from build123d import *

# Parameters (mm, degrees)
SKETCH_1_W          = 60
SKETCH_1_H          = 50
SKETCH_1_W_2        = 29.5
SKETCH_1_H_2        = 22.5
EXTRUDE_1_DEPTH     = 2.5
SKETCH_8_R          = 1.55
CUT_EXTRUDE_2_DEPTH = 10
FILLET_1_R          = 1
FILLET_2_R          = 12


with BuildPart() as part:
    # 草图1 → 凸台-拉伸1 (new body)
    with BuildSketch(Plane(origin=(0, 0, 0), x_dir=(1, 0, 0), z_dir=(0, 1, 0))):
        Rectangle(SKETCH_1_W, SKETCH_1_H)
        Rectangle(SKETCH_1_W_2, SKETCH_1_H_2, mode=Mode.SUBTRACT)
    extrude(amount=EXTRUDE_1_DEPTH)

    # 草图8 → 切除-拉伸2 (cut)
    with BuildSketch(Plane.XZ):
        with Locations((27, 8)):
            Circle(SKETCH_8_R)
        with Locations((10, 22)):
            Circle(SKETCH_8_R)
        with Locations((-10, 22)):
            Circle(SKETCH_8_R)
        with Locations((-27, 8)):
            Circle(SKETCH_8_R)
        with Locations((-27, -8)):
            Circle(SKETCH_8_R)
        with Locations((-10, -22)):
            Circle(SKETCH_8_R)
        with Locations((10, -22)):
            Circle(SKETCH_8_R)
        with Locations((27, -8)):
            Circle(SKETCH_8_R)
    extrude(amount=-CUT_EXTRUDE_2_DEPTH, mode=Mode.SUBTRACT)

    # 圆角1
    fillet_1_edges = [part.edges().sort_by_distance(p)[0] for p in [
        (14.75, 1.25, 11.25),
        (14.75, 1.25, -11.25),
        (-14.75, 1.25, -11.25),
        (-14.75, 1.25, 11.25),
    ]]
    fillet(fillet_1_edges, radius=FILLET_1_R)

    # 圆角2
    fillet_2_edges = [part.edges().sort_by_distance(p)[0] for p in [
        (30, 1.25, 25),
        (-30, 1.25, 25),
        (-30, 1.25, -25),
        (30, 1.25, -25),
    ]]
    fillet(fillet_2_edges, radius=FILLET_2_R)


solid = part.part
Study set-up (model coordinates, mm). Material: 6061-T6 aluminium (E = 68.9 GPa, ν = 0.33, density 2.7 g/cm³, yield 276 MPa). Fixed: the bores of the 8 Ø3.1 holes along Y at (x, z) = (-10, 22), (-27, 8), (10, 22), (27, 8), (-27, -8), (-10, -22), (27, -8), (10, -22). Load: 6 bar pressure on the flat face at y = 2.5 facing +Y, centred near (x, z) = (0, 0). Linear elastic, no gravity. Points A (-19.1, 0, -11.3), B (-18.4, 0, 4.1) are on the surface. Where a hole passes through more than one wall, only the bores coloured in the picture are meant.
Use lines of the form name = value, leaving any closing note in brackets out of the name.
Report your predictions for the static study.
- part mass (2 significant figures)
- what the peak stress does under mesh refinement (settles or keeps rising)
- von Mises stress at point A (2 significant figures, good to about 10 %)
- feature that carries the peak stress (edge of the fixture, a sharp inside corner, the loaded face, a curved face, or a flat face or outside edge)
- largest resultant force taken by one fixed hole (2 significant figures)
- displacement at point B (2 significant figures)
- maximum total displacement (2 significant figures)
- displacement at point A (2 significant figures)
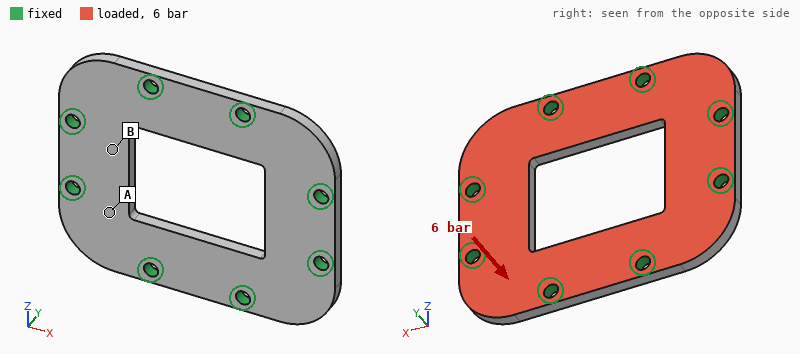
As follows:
part mass = 15 g
what the peak stress does under mesh refinement = keeps rising
von Mises stress at point A = 15 MPa
feature that carries the peak stress = edge of the fixture
largest resultant force taken by one fixed hole = 170 N
displacement at point B = 8.5 µm
maximum total displacement = 14 µm
displacement at point A = 6.0 µm
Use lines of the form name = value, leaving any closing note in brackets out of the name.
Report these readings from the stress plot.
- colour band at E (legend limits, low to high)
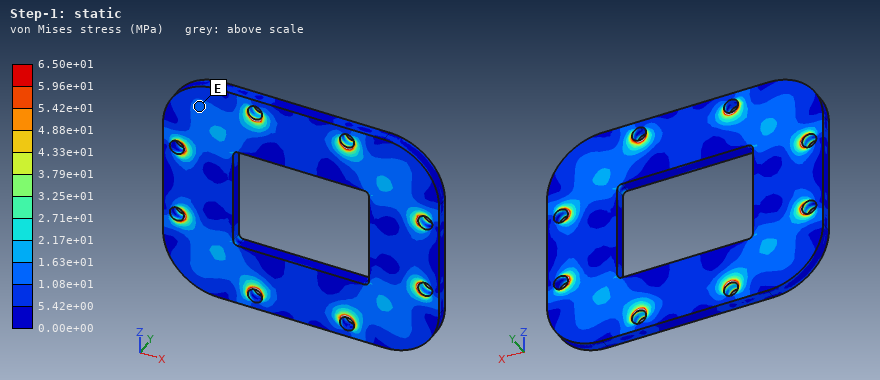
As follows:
colour band at E = 1.08e+01 to 1.63e+01 MPa
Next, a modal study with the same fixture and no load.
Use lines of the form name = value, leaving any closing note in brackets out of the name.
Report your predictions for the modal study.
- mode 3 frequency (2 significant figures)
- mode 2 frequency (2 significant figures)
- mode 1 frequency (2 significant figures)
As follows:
mode 3 frequency = 17 kHz
mode 2 frequency = 17 kHz
mode 1 frequency = 15 kHz
